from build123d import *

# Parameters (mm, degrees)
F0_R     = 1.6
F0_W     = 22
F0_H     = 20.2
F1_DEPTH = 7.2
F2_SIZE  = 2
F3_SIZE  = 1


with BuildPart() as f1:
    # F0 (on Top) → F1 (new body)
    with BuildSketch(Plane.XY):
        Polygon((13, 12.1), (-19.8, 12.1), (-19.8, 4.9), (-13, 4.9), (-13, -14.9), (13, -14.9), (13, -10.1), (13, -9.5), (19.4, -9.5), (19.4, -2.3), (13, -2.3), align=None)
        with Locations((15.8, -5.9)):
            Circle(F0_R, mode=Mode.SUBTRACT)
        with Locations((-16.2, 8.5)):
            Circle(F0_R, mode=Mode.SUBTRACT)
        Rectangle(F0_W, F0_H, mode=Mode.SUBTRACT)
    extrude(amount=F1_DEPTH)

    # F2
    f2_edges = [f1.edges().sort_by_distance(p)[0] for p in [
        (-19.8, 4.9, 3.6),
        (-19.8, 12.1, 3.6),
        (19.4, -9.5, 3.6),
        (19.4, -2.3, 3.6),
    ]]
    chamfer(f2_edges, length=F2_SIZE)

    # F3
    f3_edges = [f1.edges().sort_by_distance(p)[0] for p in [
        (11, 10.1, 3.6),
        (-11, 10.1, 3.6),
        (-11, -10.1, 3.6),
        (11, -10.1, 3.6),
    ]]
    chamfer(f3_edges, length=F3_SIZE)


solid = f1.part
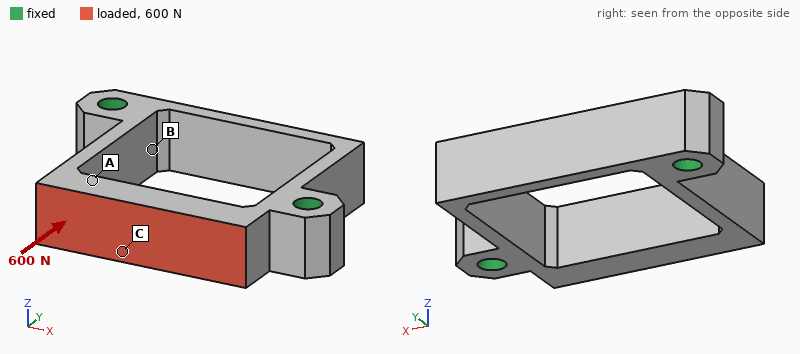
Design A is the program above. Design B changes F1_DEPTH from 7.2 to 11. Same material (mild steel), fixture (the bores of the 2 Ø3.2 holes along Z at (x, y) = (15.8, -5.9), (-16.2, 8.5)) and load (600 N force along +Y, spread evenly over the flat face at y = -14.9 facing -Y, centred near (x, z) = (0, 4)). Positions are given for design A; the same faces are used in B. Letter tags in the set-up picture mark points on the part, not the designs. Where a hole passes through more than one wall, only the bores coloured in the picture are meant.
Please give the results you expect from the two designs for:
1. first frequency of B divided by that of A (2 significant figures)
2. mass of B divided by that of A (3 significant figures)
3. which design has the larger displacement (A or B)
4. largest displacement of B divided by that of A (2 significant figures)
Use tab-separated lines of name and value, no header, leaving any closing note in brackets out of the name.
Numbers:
first frequency of B divided by that of A	1.3
mass of B divided by that of A	1.53
which design has the larger displacement	A
largest displacement of B divided by that of A	0.65
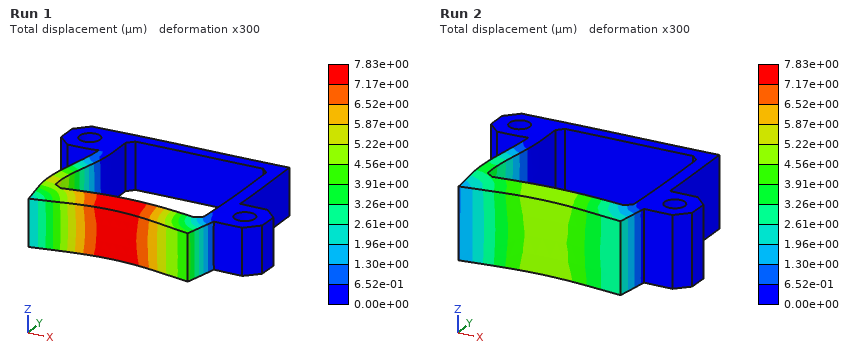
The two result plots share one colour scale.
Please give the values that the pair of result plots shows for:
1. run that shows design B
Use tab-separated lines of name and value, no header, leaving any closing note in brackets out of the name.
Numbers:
run that shows design B	Run 2
